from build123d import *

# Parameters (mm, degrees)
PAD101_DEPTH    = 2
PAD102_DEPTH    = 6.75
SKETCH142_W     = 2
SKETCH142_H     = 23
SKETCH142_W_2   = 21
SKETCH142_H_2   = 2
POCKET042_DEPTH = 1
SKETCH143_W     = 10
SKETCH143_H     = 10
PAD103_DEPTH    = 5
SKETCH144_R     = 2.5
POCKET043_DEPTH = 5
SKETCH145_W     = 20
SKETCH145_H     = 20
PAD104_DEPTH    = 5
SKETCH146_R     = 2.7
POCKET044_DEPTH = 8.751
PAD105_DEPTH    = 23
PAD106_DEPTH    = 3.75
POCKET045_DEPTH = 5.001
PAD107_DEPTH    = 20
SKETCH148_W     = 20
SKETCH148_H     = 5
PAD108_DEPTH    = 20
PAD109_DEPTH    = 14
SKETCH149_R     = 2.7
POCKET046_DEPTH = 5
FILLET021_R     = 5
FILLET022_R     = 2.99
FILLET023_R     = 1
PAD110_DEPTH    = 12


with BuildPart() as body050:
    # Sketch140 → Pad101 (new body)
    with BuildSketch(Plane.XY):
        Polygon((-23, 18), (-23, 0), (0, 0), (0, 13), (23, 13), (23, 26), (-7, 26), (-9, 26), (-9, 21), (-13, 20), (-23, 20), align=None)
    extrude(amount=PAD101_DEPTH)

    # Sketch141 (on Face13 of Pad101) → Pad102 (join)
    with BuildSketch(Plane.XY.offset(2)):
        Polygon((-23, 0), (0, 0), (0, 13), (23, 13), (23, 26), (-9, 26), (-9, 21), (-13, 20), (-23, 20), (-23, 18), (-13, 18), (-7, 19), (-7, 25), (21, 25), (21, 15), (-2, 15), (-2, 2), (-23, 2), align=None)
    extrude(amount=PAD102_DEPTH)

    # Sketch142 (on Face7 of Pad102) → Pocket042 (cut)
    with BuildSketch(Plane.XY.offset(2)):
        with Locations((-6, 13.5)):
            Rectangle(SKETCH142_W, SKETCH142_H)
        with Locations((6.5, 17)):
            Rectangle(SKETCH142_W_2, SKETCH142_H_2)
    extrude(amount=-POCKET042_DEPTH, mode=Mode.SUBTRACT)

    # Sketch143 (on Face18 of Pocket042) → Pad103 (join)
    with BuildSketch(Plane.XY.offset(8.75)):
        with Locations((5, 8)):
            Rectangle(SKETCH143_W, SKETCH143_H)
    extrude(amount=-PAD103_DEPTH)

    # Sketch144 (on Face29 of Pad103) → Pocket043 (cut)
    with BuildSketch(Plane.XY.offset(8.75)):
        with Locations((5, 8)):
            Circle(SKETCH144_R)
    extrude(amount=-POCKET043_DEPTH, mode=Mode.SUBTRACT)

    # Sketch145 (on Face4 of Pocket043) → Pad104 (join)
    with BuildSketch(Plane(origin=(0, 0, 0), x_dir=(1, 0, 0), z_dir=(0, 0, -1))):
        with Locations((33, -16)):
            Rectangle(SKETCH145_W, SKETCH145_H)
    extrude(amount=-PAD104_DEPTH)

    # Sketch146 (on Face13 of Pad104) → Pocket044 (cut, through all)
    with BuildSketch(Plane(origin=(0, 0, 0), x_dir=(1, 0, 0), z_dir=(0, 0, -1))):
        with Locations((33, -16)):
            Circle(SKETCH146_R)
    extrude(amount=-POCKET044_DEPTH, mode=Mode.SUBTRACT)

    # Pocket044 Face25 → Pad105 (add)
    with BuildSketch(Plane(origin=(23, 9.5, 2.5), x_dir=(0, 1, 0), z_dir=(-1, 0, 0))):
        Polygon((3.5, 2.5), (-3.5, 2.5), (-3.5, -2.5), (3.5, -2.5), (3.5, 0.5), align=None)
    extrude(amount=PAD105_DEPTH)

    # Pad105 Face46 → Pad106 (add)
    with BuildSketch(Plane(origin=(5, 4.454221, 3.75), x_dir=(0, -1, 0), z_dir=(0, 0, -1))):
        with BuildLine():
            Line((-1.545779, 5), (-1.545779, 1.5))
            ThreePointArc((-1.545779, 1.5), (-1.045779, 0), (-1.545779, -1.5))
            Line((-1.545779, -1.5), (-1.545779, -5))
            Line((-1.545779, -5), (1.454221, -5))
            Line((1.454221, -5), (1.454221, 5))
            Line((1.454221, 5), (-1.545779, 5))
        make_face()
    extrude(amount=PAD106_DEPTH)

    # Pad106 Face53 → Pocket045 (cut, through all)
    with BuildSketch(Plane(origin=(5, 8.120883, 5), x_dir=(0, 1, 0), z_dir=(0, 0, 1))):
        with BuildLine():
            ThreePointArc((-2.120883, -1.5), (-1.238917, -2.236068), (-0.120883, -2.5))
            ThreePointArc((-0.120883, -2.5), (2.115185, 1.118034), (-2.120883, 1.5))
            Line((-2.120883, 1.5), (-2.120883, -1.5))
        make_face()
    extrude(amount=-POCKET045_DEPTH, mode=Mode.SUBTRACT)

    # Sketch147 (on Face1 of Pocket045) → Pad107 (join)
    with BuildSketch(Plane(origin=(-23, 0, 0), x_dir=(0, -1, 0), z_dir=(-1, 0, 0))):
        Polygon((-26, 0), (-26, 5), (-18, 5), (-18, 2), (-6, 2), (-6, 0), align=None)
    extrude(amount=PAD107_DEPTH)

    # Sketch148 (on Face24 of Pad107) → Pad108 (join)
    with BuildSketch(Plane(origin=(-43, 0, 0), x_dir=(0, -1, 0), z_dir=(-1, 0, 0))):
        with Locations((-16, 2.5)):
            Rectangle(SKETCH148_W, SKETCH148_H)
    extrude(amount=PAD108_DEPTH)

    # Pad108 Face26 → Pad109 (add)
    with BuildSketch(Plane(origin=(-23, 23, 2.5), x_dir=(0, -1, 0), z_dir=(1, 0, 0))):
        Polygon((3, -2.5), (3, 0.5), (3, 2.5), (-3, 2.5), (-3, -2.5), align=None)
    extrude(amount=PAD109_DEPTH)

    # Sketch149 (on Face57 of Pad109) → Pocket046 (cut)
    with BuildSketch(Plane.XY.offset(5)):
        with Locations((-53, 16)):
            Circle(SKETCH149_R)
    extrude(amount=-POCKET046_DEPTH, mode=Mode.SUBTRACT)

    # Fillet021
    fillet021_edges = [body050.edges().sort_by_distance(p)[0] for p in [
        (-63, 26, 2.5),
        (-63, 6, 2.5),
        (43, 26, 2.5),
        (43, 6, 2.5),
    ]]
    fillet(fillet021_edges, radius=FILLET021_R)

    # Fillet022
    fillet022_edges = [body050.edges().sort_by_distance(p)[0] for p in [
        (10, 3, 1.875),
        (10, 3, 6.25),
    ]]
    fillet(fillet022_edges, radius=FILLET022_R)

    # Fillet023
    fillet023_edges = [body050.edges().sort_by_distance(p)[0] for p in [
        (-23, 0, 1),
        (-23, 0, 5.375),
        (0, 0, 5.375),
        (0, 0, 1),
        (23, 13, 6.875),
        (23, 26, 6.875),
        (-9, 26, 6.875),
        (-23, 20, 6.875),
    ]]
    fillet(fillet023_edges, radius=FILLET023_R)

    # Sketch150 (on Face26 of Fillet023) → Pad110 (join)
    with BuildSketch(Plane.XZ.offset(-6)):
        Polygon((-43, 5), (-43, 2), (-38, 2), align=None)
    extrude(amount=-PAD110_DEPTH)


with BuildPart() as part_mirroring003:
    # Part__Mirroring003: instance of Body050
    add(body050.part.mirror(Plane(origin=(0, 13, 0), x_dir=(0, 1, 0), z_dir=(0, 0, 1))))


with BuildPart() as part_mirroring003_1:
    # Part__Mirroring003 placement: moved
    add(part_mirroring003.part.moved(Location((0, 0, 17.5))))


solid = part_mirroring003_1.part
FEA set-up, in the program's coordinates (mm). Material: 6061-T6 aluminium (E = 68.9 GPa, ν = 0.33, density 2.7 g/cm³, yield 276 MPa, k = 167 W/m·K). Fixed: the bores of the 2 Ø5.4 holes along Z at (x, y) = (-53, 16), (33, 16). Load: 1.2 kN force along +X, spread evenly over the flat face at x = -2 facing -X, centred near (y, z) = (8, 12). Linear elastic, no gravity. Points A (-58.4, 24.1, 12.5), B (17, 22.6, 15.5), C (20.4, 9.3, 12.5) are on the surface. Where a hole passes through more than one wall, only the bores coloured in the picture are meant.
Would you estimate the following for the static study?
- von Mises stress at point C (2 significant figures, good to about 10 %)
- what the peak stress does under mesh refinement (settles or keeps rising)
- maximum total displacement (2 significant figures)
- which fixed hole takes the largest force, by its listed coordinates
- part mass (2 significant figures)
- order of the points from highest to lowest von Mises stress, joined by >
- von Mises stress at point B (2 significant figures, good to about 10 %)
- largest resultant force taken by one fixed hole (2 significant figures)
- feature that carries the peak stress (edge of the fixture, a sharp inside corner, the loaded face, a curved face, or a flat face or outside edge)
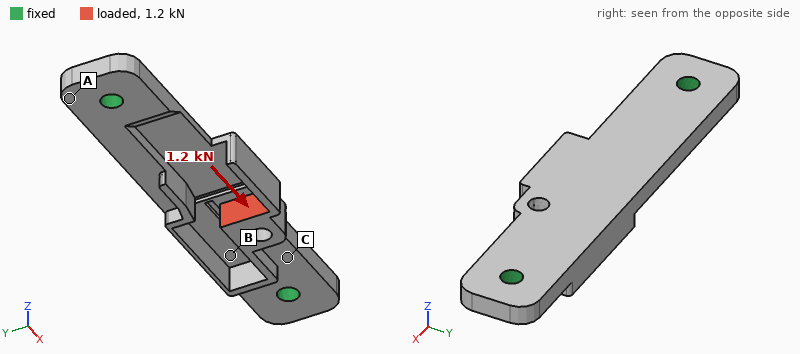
32 MPa
keeps rising
91 µm
(33, 16)
26 g
C > B > A
11 MPa
1.0 kN
a sharp inside corner
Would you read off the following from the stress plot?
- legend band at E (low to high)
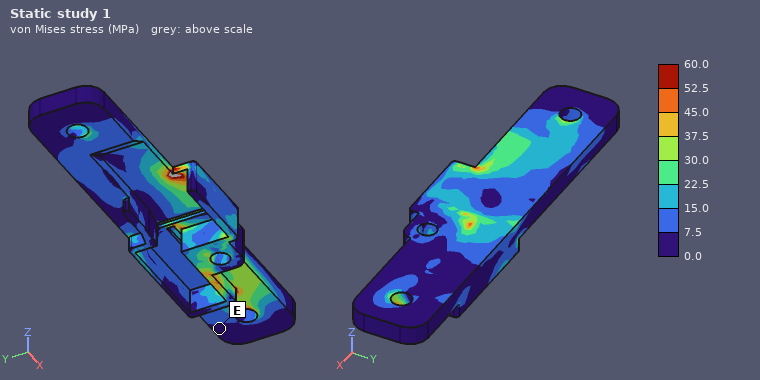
0.0 to 7.5 MPa
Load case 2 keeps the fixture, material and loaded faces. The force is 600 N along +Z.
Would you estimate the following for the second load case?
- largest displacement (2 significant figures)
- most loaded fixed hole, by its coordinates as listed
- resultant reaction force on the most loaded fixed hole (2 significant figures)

0.34 mm
(33, 16)
610 N
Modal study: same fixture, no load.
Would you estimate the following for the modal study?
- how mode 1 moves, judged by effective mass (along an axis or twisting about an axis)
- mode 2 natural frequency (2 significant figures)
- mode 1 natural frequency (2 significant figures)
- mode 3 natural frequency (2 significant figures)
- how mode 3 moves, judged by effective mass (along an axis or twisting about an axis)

along Z
5100 Hz
3000 Hz
8000 Hz
along Y
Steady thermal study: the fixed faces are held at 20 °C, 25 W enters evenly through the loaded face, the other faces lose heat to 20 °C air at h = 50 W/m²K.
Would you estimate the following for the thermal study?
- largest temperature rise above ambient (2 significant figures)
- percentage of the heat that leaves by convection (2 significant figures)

42 K
20 %
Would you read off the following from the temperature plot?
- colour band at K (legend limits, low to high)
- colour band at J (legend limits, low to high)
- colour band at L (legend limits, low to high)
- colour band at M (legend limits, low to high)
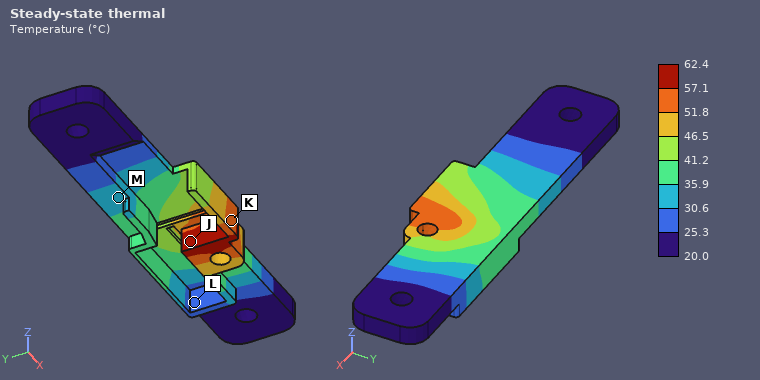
51.8 to 57.1 °C
57.1 to 62.4 °C
25.3 to 30.6 °C
30.6 to 35.9 °C
